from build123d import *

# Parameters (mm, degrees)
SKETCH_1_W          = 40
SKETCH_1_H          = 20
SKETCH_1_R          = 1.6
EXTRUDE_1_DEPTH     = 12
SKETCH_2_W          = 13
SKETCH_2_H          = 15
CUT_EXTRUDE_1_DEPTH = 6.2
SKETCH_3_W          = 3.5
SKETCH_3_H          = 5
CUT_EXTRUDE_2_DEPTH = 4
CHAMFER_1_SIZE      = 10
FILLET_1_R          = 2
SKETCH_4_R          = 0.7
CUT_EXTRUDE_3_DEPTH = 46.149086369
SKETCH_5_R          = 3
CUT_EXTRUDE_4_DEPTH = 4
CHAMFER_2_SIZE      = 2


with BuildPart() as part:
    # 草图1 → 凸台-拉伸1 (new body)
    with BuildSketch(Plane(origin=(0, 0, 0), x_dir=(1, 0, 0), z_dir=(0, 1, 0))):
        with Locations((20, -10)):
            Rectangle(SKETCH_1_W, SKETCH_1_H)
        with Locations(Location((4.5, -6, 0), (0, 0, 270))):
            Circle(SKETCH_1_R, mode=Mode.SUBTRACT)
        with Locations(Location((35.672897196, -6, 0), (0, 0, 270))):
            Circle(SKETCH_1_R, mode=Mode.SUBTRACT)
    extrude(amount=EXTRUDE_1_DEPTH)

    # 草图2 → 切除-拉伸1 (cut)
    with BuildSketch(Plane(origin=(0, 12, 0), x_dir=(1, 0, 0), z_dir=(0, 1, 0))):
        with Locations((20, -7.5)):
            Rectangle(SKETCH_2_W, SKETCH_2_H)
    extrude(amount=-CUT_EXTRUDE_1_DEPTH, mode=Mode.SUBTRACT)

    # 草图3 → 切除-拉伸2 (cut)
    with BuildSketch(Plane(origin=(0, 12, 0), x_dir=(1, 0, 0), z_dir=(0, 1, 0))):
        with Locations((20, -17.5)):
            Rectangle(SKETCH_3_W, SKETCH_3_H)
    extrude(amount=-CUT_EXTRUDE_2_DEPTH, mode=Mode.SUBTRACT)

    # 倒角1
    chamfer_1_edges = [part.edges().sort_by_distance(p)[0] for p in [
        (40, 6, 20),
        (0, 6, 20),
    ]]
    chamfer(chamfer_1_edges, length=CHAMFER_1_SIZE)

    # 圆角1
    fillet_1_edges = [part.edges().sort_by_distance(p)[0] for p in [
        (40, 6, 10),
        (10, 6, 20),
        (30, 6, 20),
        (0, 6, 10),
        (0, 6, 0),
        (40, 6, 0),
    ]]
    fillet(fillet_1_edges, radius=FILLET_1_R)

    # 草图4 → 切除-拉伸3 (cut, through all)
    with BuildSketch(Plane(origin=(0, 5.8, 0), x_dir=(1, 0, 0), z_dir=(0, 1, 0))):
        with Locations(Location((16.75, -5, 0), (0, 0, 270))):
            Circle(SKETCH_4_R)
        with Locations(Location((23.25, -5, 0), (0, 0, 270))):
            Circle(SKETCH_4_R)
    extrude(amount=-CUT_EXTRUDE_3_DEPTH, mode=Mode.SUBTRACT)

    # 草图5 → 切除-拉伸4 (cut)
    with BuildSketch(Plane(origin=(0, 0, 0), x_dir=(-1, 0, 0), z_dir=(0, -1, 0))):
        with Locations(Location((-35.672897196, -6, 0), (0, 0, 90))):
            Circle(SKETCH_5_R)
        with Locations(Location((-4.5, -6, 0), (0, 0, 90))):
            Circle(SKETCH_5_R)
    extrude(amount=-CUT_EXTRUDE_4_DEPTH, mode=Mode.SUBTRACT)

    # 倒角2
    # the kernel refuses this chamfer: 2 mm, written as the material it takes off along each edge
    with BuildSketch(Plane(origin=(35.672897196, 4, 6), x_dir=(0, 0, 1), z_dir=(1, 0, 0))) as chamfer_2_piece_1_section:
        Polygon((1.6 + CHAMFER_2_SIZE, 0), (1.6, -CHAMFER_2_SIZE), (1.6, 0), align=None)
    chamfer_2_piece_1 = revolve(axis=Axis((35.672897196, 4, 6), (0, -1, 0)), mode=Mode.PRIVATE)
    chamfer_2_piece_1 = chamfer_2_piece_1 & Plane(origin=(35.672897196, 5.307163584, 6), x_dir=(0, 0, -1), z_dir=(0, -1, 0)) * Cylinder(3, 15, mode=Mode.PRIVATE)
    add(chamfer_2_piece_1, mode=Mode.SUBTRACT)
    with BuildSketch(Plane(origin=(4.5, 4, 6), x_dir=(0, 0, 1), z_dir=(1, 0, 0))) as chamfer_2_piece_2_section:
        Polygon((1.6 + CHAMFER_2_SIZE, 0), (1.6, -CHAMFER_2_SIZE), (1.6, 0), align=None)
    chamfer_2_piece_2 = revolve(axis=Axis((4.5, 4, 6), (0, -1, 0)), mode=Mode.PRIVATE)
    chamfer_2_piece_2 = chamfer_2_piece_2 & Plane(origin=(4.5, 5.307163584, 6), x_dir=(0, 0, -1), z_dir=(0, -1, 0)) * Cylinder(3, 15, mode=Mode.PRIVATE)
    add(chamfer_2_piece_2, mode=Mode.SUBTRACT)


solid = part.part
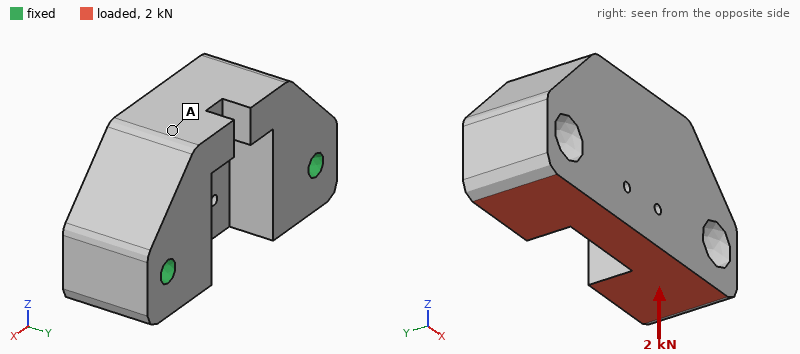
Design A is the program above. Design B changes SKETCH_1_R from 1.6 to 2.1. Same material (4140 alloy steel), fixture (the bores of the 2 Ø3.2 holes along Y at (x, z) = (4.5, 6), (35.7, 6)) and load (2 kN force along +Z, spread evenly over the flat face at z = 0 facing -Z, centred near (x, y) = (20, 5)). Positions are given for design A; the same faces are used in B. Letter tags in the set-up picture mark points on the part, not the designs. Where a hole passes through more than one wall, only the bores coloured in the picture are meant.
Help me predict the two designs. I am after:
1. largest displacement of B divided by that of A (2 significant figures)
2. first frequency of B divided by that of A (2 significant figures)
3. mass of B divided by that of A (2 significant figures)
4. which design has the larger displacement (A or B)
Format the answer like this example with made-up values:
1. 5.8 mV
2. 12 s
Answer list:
1. 0.69
2. 1.2
3. 0.99
4. A
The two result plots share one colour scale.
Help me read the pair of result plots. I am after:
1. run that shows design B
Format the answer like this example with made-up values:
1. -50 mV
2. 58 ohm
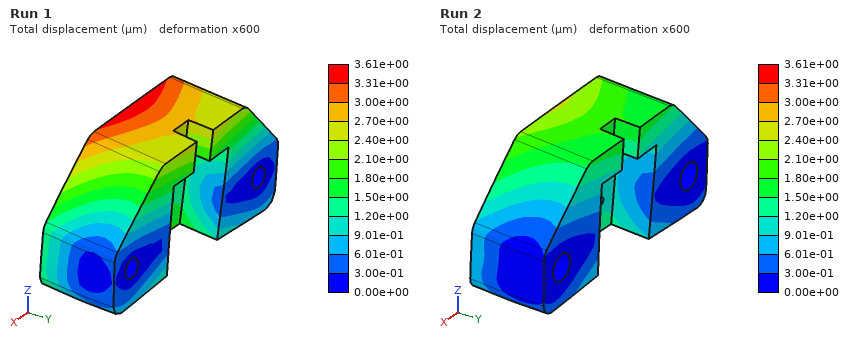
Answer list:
1. Run 2
